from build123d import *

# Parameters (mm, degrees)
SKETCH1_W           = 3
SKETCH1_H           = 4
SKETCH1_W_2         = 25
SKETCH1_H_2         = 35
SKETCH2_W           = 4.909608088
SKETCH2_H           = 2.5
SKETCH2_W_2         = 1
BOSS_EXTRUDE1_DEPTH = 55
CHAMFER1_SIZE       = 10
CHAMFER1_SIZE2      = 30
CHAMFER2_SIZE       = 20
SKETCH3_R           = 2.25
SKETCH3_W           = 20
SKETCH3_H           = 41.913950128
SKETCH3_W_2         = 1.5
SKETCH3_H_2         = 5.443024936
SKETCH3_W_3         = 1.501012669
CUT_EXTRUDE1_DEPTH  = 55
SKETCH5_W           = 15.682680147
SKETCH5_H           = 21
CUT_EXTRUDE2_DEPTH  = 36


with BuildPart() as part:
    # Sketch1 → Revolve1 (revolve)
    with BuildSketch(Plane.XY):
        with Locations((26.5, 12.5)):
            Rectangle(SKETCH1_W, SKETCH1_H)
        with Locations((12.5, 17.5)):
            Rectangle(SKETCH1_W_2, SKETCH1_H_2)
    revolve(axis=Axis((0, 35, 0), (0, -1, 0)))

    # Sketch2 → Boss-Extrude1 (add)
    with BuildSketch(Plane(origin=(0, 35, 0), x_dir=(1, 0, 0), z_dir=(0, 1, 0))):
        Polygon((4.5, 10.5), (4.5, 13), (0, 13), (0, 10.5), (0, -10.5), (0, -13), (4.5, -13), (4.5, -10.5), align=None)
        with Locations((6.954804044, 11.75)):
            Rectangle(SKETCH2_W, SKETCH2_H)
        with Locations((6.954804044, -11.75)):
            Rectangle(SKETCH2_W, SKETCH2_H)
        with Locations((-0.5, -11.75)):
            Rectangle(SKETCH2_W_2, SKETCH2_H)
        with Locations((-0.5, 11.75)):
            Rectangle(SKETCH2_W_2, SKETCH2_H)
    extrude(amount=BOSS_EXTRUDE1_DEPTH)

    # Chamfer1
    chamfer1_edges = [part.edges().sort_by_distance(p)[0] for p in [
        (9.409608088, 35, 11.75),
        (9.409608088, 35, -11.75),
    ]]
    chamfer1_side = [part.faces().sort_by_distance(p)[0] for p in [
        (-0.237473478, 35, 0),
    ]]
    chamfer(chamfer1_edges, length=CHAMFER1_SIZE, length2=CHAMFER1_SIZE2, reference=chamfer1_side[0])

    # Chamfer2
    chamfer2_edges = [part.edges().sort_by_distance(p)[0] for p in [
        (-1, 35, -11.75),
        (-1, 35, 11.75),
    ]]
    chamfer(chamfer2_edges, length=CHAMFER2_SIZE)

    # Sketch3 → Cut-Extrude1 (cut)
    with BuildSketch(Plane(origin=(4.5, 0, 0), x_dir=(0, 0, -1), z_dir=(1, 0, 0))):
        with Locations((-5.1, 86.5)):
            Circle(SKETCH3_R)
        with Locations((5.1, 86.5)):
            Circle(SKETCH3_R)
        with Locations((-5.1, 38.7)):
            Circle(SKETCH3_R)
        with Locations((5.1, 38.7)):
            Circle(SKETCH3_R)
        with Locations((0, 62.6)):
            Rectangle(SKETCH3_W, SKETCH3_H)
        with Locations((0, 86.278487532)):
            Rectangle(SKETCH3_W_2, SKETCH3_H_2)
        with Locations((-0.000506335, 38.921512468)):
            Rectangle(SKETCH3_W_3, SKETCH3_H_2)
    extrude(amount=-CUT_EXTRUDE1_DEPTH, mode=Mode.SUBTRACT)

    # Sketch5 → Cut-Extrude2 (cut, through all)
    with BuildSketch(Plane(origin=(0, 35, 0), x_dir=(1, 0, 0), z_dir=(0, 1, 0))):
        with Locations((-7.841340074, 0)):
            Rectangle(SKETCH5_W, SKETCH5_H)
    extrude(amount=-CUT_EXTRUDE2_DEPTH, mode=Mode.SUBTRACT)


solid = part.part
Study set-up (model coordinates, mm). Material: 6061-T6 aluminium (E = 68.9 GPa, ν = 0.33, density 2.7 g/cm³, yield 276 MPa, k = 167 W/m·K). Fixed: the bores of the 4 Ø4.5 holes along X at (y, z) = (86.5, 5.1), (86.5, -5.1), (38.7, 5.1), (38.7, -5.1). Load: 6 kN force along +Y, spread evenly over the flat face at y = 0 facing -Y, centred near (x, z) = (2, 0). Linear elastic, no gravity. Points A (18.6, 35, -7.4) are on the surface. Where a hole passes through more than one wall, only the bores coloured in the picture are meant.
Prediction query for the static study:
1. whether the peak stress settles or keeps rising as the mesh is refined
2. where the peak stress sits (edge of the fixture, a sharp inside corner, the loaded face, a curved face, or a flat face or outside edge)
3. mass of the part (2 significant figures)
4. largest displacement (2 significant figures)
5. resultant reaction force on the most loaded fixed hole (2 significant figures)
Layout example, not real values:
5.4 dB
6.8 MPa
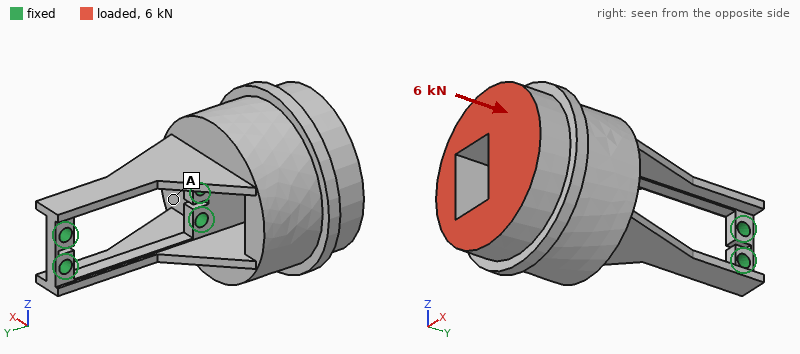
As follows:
keeps rising
edge of the fixture
180 g
30 µm
2.9 kN
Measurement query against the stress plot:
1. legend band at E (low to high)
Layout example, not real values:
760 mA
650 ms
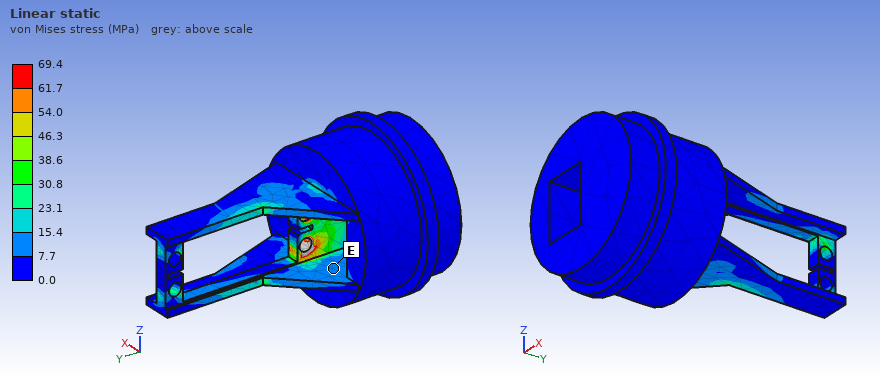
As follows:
7.7 to 15.4 MPa
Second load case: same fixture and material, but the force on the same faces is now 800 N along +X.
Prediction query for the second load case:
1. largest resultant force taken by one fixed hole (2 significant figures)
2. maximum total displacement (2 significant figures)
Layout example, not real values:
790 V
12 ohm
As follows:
660 N
0.12 mm
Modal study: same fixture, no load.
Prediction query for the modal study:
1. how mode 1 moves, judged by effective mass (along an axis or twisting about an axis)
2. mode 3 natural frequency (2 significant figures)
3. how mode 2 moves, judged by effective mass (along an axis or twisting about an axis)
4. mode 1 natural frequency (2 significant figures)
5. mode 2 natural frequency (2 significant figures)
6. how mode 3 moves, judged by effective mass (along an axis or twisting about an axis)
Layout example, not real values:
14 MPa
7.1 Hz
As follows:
along X
3200 Hz
along Z
1700 Hz
2600 Hz
along Z
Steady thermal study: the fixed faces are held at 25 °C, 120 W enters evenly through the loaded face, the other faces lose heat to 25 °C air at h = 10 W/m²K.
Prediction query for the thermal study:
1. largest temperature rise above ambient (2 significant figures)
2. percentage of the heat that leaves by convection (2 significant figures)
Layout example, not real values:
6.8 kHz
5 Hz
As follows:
50 K
4.3 %
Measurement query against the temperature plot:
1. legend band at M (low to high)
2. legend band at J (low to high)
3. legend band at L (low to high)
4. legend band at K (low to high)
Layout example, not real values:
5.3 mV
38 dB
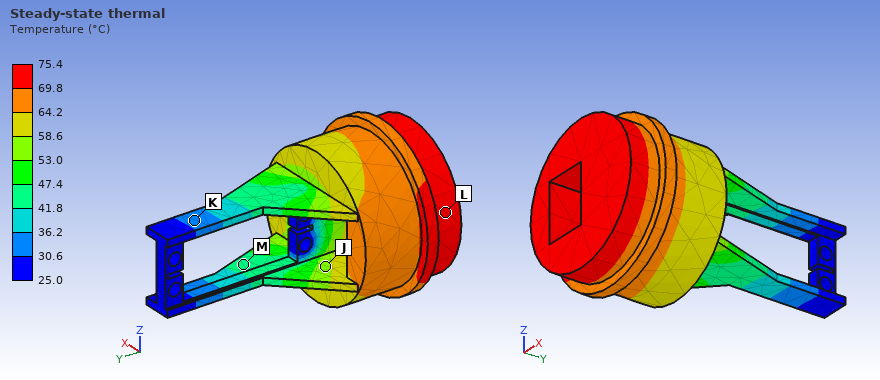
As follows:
41.8 to 47.4 °C
53.0 to 58.6 °C
69.8 to 75.4 °C
30.6 to 36.2 °C
